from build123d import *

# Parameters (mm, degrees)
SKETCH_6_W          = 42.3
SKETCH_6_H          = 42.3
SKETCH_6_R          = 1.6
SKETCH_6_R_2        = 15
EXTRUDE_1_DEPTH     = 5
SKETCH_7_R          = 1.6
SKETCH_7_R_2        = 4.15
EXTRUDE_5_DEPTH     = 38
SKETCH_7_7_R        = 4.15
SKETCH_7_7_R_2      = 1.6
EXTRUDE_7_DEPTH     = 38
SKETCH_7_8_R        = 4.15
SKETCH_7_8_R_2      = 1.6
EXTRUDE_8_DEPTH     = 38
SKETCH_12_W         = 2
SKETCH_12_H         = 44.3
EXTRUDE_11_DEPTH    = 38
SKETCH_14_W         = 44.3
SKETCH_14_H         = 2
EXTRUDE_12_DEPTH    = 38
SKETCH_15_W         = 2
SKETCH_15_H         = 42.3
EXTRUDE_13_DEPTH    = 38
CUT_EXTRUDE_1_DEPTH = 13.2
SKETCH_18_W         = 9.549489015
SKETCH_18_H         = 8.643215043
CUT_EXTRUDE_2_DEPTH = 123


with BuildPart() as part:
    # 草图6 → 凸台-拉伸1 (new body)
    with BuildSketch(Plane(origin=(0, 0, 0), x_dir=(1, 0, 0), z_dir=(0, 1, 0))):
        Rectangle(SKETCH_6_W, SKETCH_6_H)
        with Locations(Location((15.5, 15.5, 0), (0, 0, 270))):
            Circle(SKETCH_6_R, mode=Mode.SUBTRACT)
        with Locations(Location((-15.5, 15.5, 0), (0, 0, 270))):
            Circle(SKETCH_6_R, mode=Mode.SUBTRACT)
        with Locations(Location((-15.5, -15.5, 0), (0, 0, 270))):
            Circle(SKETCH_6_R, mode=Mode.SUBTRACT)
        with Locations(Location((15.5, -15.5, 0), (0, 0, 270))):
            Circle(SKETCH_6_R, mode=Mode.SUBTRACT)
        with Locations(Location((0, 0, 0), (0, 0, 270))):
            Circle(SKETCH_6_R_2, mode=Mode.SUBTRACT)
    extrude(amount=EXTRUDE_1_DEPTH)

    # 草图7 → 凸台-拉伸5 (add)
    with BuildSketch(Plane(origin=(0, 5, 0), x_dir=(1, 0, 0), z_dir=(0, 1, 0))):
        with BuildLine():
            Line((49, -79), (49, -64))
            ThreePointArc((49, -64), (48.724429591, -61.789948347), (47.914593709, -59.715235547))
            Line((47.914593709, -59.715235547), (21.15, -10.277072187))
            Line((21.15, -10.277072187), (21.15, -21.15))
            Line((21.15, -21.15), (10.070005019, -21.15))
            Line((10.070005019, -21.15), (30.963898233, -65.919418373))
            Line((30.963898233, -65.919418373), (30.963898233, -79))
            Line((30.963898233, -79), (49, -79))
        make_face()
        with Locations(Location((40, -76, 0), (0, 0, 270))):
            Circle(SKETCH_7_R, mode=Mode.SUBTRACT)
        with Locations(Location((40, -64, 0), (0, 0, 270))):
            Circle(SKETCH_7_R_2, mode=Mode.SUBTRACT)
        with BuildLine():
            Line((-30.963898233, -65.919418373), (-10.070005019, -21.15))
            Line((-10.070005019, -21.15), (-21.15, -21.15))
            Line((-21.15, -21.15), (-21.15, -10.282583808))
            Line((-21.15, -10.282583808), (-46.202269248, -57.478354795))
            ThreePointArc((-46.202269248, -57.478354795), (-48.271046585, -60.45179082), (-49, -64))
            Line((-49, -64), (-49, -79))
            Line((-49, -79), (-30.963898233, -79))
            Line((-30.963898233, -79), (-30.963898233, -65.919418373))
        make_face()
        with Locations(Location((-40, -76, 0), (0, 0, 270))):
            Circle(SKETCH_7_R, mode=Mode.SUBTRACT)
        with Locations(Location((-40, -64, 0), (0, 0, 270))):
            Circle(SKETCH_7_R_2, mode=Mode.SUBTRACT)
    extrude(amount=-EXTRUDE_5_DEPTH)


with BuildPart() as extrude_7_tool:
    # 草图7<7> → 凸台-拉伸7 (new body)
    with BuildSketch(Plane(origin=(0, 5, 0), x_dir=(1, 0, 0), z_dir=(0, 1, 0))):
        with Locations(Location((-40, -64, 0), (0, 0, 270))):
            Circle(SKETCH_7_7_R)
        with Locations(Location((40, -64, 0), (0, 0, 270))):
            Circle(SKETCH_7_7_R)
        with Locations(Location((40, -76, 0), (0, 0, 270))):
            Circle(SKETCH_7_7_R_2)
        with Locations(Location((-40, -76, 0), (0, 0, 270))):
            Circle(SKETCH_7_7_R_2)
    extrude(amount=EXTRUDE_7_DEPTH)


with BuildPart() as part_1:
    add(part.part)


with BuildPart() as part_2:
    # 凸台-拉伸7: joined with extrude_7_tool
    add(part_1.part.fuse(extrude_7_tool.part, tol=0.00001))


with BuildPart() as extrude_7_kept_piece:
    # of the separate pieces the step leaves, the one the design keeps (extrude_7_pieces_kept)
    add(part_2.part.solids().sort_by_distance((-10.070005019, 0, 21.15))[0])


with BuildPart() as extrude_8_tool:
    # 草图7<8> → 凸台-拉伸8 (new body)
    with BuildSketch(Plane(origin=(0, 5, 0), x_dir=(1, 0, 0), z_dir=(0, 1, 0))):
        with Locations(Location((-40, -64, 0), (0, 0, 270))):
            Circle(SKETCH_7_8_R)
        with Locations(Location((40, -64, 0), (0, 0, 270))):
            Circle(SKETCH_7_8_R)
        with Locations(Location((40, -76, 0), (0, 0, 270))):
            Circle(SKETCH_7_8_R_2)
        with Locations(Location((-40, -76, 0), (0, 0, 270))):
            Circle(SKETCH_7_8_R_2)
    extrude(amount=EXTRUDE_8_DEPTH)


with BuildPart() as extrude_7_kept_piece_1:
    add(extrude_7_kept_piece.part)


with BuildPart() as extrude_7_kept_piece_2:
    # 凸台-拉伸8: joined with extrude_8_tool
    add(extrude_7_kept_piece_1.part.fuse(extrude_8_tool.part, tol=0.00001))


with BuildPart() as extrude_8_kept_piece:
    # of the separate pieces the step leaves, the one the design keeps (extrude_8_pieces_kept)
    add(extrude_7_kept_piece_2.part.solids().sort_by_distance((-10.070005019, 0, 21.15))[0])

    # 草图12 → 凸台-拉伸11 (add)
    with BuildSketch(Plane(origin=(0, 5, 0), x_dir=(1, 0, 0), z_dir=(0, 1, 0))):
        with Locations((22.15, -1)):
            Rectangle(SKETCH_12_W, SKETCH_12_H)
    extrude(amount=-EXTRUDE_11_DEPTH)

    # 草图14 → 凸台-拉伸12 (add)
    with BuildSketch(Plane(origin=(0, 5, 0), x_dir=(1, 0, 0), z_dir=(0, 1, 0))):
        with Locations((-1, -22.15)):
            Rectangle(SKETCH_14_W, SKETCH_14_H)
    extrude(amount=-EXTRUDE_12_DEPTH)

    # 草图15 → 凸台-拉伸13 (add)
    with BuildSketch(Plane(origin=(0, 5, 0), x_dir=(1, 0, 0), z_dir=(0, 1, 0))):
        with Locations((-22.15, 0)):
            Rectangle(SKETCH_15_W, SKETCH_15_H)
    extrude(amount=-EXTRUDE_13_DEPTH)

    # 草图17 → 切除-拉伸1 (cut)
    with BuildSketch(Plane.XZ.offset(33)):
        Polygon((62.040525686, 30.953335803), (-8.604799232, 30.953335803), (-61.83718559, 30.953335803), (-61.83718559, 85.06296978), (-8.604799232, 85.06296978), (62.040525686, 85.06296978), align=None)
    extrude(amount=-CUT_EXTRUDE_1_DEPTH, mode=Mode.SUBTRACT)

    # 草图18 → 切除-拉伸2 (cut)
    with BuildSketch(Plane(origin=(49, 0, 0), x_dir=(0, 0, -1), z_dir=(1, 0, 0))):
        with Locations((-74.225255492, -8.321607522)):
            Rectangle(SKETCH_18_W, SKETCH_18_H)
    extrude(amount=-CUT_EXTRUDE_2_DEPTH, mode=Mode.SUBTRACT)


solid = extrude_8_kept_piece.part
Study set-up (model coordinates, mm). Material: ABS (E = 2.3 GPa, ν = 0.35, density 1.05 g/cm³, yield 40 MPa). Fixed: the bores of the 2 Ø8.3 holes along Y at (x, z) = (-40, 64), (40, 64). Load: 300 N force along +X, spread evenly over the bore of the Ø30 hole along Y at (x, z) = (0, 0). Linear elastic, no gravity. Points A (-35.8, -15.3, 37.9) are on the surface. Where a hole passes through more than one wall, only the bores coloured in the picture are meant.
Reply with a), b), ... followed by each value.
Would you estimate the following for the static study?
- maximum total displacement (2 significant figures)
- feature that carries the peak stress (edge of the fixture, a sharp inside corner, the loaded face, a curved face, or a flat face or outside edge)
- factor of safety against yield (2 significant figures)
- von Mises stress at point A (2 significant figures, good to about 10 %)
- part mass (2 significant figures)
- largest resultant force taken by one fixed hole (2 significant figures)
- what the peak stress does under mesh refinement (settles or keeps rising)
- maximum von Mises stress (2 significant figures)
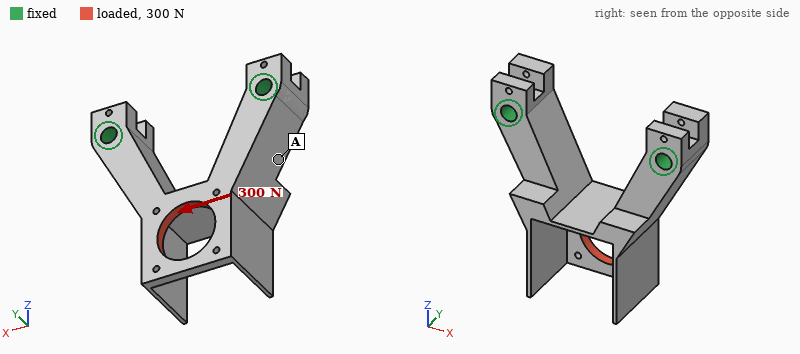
a) 0.38 mm
b) the loaded face
c) 3.2
d) 1.4 MPa
e) 69 g
f) 240 N
g) settles
h) 13 MPa
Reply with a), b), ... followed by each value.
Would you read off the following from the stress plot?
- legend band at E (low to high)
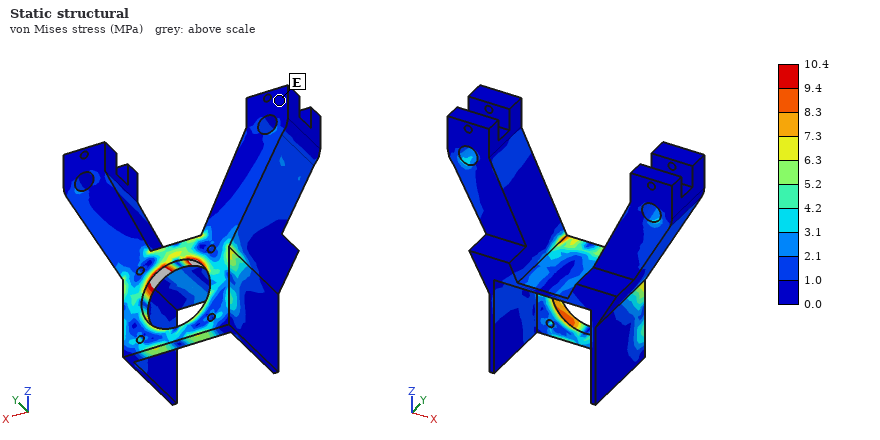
a) 0.0 to 1.0 MPa
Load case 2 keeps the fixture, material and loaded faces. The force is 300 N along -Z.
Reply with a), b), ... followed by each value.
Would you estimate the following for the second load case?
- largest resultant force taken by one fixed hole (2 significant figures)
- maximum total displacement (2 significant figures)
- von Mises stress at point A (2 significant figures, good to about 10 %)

a) 160 N
b) 0.16 mm
c) 0.30 MPa
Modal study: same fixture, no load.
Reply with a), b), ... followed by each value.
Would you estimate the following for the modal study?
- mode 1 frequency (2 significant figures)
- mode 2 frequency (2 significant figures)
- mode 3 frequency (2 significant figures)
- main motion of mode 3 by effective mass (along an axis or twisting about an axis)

a) 710 Hz
b) 730 Hz
c) 1000 Hz
d) along Y
